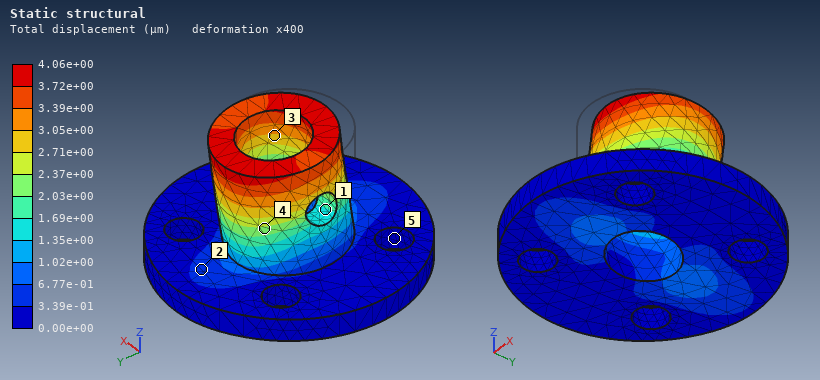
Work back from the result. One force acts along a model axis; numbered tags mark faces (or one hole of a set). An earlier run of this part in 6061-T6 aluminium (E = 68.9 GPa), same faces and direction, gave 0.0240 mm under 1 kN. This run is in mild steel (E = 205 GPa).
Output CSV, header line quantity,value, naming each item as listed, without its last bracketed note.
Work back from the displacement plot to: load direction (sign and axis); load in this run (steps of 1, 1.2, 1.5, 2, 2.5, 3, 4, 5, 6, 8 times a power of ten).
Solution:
quantity,value
load direction,+Y
load in this run,500 N
